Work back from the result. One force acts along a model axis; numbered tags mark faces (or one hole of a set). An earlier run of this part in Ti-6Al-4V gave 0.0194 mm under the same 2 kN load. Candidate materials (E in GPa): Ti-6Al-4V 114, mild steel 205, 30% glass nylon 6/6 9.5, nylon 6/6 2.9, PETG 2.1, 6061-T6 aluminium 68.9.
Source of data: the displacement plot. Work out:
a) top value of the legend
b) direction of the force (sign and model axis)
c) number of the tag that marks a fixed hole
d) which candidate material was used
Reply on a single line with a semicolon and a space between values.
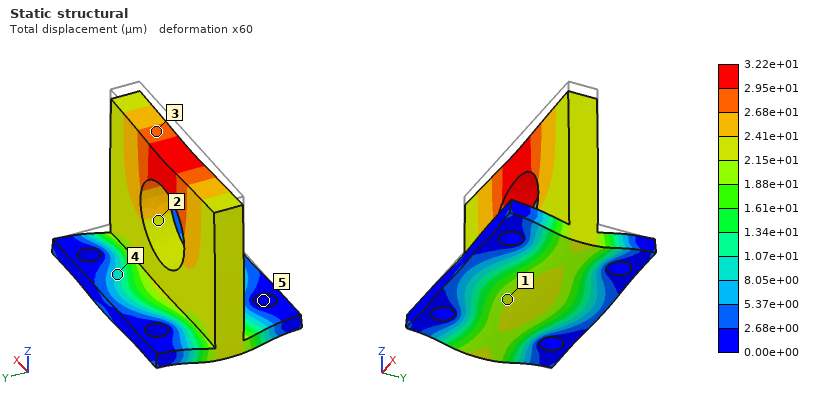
3.22e+01 µm; -Z; 5; 6061-T6 aluminium
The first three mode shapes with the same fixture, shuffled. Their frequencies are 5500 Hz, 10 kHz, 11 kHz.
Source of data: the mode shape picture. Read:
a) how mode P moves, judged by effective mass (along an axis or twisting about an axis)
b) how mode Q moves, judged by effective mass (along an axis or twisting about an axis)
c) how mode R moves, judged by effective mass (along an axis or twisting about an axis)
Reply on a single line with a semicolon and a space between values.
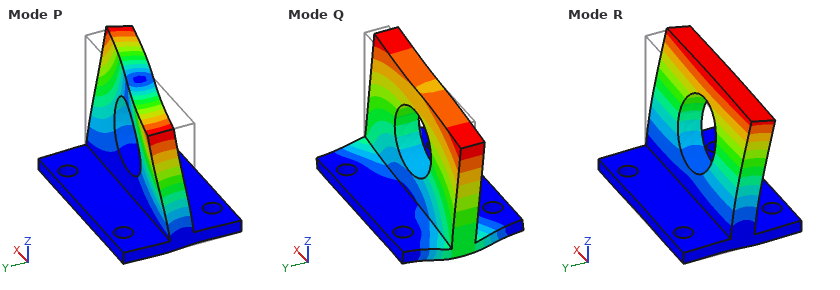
twisting about Z; along X; along Y
